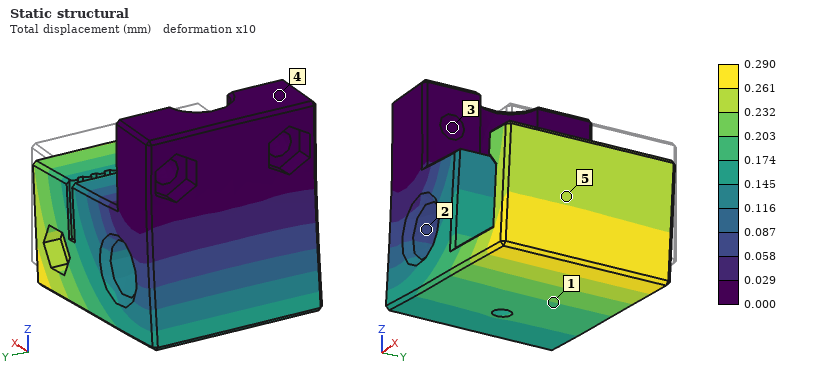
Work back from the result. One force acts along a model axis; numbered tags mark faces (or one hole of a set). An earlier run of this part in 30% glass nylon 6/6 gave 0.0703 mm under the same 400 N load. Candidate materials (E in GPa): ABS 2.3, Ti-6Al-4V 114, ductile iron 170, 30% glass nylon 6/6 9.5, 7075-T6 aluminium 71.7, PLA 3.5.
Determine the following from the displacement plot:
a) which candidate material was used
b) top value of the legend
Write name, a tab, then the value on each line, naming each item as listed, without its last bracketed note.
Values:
which candidate material was used	ABS
top value of the legend	0.290 mm
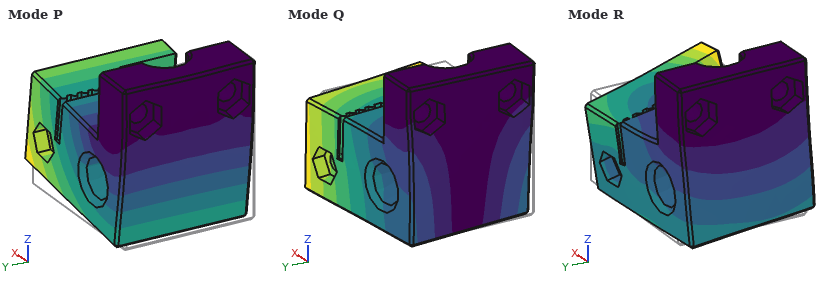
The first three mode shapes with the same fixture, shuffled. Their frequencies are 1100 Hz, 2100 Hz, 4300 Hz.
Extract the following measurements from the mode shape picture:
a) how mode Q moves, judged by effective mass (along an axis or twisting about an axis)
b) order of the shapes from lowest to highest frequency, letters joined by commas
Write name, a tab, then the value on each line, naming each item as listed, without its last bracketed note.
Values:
how mode Q moves, judged by effective mass	along Y
order of the shapes from lowest to highest frequency, letters joined by commas	P, Q, R
